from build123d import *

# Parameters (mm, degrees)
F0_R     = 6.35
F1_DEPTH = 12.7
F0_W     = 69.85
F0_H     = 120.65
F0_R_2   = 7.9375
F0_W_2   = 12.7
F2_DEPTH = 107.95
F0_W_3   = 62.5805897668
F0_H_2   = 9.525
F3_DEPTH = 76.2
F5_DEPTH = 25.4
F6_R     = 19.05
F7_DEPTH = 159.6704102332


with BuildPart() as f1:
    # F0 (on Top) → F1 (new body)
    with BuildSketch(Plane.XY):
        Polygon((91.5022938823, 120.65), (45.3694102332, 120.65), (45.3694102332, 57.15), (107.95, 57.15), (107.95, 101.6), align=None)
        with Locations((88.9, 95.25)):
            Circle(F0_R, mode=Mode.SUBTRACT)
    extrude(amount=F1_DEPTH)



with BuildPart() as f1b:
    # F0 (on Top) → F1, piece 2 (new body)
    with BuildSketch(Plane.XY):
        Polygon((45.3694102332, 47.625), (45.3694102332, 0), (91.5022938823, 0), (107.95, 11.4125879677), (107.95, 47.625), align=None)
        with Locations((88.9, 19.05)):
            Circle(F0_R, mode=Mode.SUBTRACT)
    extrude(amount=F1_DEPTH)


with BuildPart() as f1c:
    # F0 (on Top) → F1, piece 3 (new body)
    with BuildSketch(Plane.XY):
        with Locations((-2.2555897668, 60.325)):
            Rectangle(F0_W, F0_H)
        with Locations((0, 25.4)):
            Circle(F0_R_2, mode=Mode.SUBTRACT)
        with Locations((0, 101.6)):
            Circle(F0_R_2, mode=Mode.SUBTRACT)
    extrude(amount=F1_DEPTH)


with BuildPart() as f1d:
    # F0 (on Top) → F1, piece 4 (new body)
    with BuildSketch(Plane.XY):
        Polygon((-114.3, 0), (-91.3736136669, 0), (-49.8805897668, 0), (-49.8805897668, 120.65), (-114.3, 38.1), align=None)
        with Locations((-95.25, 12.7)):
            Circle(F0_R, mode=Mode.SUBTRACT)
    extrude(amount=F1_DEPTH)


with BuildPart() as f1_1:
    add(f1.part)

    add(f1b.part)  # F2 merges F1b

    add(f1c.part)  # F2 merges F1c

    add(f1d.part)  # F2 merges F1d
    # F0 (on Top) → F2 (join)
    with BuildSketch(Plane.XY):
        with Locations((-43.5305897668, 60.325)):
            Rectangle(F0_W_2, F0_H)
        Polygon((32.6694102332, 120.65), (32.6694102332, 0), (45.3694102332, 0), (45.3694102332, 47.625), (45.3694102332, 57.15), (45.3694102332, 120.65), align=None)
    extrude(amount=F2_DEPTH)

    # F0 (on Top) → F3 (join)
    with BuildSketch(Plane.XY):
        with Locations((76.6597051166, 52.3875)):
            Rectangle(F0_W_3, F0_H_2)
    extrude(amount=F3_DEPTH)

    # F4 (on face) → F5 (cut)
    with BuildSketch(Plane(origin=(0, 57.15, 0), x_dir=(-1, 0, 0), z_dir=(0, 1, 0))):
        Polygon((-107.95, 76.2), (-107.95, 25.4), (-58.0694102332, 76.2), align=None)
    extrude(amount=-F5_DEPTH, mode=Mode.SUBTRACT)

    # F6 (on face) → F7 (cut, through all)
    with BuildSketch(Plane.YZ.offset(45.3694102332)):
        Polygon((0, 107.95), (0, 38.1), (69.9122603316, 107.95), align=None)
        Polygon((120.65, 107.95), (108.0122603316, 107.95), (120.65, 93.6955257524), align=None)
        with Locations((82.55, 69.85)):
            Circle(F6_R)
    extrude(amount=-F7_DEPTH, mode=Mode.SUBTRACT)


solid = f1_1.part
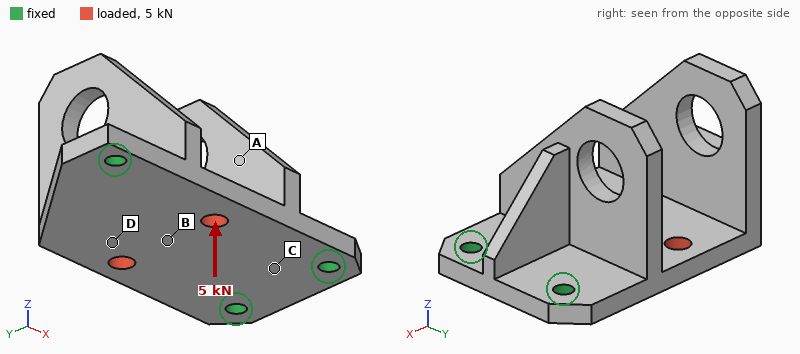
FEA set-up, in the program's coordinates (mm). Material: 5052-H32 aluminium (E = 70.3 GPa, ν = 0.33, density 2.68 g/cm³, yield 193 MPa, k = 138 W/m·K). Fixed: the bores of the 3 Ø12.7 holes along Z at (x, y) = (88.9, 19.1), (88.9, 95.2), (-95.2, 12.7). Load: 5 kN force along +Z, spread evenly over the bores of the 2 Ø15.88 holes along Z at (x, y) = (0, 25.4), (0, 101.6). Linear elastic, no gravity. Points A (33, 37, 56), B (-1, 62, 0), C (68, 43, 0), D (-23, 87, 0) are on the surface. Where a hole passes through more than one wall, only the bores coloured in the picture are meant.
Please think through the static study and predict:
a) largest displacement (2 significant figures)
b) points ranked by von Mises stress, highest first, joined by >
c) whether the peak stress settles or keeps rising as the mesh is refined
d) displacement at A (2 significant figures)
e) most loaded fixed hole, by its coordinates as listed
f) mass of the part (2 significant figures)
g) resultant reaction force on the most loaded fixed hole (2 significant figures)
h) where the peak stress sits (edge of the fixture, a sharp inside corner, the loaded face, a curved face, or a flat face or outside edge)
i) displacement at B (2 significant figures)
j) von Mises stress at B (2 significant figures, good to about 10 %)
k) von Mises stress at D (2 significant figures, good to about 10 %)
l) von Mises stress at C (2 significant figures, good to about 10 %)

0.30 mm
B > D > C > A
keeps rising
0.13 mm
(88.9, 95.2)
1.4 kg
2.4 kN
edge of the fixture
0.16 mm
29 MPa
21 MPa
12 MPa
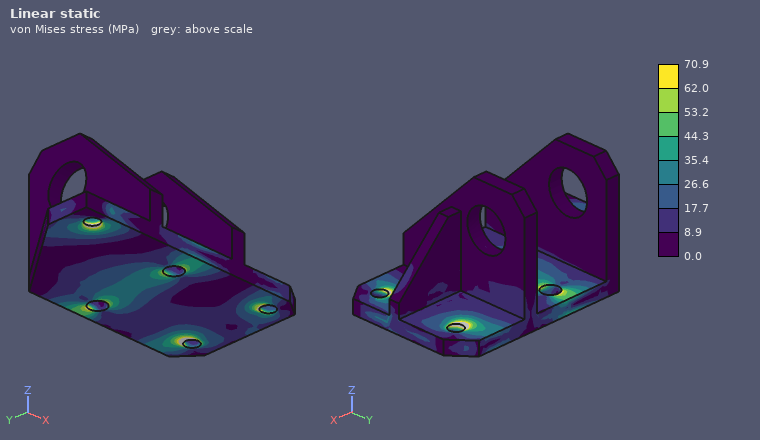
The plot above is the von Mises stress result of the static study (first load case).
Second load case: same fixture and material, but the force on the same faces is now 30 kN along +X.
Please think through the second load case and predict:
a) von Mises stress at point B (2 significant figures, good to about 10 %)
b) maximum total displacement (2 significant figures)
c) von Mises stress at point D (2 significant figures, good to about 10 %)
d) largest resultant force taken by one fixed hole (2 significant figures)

6.2 MPa
30 µm
12 MPa
11 kN
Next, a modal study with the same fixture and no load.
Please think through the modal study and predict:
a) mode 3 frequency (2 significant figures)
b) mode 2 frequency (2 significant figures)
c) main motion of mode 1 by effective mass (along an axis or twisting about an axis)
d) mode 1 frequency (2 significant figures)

1500 Hz
1000 Hz
along Z
780 Hz
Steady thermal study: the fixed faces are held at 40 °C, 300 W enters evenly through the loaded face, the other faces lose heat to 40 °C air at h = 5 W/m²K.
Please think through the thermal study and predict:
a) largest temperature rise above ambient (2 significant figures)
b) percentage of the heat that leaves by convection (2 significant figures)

89 K
6.7 %
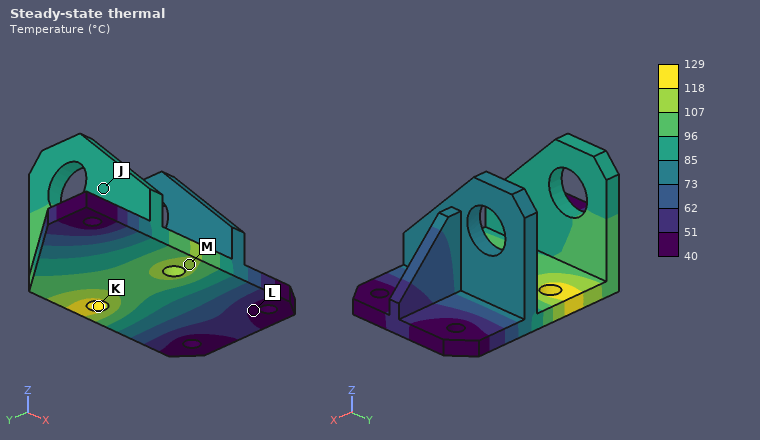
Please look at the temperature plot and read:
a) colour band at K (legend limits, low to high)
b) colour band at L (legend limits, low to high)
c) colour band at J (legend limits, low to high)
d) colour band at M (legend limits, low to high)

118 to 129 °C
40 to 51 °C
85 to 96 °C
107 to 118 °C
